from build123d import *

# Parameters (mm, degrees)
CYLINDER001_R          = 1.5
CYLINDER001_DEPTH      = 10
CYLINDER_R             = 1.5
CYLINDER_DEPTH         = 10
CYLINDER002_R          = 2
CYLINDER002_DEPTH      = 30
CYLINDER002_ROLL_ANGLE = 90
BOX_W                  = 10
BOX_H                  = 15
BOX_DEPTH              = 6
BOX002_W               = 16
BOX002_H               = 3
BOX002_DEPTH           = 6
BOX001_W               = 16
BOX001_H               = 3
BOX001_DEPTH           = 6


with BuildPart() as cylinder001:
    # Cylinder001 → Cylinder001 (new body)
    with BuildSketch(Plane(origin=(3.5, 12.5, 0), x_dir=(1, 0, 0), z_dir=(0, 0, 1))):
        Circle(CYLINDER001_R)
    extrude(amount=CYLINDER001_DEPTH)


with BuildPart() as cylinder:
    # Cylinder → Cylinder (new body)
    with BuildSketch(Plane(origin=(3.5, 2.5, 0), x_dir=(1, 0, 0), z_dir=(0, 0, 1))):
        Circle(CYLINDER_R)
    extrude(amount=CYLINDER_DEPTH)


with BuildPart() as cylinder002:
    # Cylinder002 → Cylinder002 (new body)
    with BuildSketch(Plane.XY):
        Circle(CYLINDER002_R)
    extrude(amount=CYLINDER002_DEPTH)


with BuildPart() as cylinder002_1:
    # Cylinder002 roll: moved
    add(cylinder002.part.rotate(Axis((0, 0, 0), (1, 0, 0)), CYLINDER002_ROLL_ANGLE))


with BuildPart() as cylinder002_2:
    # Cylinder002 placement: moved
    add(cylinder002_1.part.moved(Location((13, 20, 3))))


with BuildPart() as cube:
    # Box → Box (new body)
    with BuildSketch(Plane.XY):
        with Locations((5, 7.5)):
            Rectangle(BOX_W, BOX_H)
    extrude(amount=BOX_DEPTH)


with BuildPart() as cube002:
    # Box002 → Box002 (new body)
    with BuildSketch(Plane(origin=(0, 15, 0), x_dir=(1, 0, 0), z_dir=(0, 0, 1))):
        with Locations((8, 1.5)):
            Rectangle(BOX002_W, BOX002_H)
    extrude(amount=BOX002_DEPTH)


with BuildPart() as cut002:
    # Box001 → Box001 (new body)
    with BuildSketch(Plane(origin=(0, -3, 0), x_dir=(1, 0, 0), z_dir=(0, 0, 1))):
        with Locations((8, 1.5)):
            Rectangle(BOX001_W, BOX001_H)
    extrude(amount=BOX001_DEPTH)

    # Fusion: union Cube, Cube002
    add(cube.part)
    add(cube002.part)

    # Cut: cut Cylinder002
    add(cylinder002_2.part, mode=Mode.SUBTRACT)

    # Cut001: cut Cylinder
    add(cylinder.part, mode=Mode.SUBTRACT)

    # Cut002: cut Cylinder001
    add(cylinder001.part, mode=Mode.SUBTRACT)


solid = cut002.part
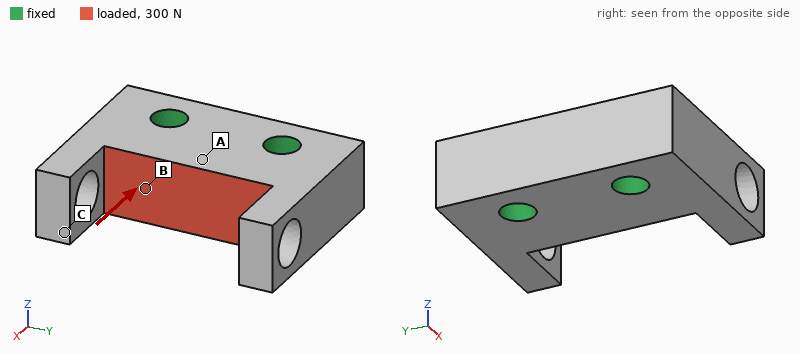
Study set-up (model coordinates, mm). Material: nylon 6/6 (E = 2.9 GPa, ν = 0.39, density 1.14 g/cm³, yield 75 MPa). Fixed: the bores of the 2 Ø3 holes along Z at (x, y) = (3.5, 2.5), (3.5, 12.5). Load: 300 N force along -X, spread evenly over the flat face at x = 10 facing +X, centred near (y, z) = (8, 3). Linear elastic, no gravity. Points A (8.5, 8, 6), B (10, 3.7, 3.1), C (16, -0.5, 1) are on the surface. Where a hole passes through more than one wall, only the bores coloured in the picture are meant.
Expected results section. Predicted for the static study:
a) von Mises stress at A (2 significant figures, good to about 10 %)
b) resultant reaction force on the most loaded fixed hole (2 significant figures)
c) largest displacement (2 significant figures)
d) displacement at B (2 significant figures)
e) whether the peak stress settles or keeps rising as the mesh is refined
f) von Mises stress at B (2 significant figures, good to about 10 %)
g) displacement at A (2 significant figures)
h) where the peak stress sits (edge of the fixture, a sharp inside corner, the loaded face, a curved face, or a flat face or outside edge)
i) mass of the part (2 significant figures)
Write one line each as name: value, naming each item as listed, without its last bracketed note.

von Mises stress at A: 2.7 MPa
resultant reaction force on the most loaded fixed hole: 150 N
largest displacement: 8.3 µm
displacement at B: 6.8 µm
whether the peak stress settles or keeps rising as the mesh is refined: keeps rising
von Mises stress at B: 3.2 MPa
displacement at A: 6.9 µm
where the peak stress sits: edge of the fixture
mass of the part: 1.5 g
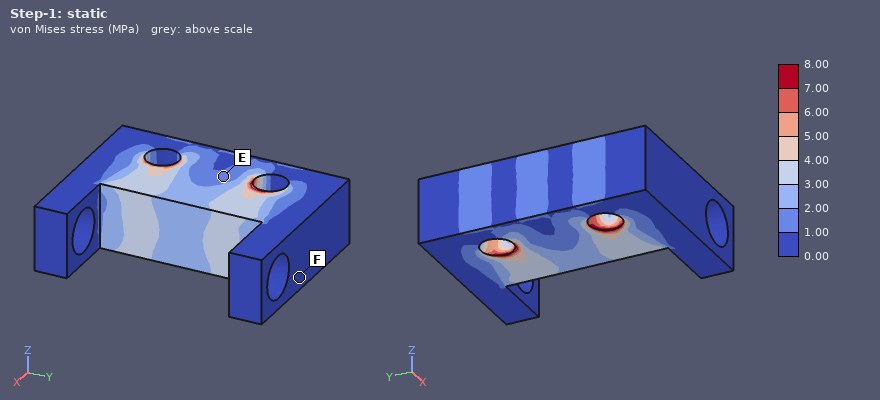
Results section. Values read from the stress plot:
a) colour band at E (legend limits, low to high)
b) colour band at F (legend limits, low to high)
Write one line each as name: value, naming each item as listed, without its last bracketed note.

colour band at E: 1.00 to 2.00 MPa
colour band at F: 0.00 to 1.00 MPa
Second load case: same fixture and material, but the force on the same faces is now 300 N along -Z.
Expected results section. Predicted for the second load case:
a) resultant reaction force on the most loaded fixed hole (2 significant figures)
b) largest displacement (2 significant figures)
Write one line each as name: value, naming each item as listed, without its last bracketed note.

resultant reaction force on the most loaded fixed hole: 150 N
largest displacement: 61 µm
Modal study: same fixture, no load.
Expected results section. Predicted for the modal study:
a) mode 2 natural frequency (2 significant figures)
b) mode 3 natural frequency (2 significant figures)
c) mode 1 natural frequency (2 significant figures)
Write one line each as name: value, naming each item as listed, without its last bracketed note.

mode 2 natural frequency: 11 kHz
mode 3 natural frequency: 11 kHz
mode 1 natural frequency: 11 kHz
